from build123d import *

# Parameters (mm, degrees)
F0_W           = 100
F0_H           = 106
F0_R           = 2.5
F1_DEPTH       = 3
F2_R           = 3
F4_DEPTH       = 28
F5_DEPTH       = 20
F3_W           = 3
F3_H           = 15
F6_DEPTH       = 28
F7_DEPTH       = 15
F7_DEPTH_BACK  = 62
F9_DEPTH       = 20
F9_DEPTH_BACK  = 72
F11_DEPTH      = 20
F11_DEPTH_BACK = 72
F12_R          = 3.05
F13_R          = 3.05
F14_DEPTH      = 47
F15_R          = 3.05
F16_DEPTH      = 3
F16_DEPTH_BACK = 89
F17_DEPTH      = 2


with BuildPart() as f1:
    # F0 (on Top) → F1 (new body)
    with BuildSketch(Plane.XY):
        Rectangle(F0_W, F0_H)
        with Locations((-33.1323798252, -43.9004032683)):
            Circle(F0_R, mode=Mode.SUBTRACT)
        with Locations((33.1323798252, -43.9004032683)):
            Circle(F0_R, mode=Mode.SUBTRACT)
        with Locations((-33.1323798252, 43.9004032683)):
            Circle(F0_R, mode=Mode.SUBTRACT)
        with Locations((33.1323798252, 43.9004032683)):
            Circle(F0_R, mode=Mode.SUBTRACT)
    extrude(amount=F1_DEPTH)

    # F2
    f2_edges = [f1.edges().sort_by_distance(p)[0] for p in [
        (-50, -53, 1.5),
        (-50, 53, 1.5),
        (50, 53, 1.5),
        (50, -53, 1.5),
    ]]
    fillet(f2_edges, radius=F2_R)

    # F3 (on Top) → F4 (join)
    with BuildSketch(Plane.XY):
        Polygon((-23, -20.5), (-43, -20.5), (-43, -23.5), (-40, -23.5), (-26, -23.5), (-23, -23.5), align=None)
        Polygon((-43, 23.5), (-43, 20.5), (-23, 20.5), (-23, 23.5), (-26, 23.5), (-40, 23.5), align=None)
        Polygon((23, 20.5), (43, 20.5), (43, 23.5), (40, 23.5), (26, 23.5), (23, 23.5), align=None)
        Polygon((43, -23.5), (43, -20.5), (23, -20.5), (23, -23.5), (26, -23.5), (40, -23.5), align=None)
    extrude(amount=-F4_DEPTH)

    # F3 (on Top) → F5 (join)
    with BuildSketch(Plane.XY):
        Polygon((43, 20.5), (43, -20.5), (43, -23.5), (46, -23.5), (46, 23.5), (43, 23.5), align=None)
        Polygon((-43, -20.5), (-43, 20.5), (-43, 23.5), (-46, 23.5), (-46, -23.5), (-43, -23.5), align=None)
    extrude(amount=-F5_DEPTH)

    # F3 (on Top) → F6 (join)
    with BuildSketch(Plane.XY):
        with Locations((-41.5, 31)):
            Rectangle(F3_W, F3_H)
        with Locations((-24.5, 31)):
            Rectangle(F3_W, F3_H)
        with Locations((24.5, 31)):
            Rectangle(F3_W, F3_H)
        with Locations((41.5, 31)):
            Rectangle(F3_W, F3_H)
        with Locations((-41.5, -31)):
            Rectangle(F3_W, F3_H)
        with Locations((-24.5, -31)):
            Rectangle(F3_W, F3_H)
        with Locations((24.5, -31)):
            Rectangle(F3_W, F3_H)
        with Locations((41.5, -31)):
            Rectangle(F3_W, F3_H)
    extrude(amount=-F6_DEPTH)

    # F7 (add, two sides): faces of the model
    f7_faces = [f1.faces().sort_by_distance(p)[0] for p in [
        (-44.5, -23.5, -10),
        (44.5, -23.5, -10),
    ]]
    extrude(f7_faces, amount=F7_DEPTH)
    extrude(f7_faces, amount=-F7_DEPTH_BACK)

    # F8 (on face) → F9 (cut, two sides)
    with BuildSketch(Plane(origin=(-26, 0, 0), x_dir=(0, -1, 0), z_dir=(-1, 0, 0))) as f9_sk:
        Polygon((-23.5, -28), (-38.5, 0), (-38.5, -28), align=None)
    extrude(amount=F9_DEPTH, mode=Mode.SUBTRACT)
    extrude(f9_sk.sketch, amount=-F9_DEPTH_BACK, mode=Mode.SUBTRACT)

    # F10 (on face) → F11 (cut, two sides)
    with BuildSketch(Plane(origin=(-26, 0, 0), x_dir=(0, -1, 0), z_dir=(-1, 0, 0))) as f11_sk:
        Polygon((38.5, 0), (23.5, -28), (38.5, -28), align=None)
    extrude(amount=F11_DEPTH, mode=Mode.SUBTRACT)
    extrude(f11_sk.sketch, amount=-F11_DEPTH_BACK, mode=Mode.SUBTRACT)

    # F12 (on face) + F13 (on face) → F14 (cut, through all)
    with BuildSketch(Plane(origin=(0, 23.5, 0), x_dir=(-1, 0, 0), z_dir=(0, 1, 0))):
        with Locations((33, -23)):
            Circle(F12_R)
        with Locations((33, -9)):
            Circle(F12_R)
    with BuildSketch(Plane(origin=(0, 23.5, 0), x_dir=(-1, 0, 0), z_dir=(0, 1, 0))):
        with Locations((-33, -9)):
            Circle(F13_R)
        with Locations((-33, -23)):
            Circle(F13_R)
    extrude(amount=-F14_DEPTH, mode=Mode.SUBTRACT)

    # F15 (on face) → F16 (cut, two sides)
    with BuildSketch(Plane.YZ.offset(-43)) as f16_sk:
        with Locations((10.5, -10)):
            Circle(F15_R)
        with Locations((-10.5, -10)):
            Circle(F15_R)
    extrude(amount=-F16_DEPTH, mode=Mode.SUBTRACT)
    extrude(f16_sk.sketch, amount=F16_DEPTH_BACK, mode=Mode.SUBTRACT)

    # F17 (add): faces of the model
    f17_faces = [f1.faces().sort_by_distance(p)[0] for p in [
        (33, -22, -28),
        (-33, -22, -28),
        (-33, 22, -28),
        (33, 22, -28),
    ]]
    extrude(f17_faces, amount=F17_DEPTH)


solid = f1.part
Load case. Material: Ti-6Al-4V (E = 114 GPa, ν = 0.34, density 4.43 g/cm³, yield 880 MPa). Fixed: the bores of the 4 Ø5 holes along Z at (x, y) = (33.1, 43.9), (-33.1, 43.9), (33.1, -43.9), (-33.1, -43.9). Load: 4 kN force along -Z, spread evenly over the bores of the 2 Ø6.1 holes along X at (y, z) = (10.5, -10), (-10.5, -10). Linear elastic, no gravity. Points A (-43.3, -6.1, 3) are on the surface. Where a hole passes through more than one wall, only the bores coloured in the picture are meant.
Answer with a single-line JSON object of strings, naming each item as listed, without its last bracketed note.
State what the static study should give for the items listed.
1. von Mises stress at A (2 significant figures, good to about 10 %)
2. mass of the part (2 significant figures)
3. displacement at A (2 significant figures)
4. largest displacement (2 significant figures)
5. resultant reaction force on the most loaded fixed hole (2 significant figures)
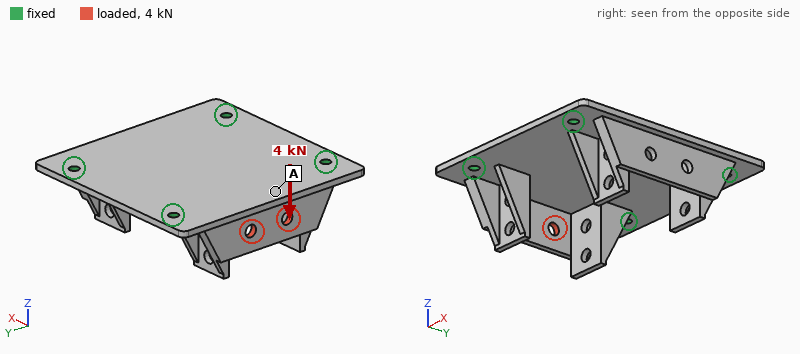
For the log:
{"von Mises stress at A": "58 MPa", "mass of the part": "220 g", "displacement at A": "0.18 mm", "largest displacement": "0.30 mm", "resultant reaction force on the most loaded fixed hole": "2.9 kN"}
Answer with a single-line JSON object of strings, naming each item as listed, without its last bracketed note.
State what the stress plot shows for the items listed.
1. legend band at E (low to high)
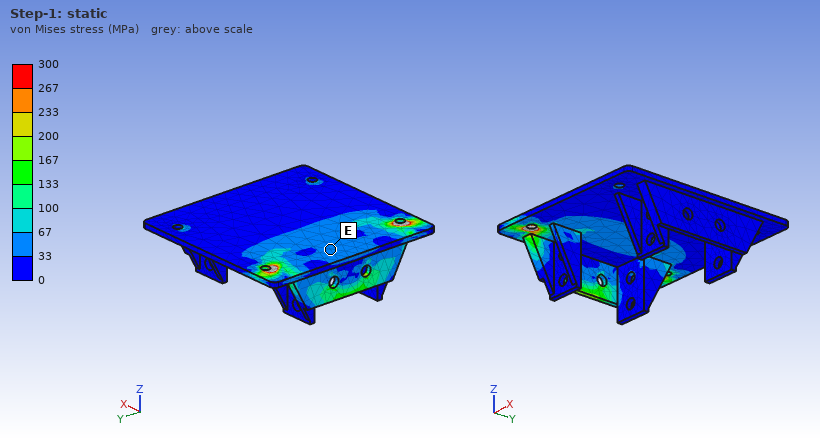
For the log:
{"legend band at E": "33 to 67 MPa"}
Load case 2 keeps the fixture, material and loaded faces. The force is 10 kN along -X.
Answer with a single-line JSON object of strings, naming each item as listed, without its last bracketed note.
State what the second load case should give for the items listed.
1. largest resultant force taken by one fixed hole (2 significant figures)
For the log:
{"largest resultant force taken by one fixed hole": "2.8 kN"}
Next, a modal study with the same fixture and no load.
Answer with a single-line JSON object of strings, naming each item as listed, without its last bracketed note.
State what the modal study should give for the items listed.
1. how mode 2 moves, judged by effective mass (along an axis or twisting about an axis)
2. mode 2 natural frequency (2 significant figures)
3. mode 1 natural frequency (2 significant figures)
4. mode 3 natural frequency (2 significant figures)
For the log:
{"how mode 2 moves, judged by effective mass": "along X", "mode 2 natural frequency": "3100 Hz", "mode 1 natural frequency": "2000 Hz", "mode 3 natural frequency": "3300 Hz"}
